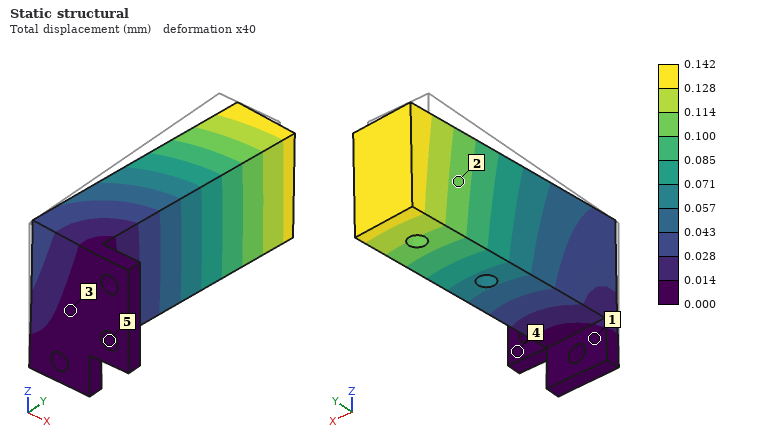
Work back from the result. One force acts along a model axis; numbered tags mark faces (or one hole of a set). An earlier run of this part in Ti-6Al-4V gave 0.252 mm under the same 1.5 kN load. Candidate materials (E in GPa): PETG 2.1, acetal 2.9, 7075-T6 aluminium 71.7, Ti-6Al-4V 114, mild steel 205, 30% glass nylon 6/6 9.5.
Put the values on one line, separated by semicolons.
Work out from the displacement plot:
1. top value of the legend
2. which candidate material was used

0.142 mm; mild steel
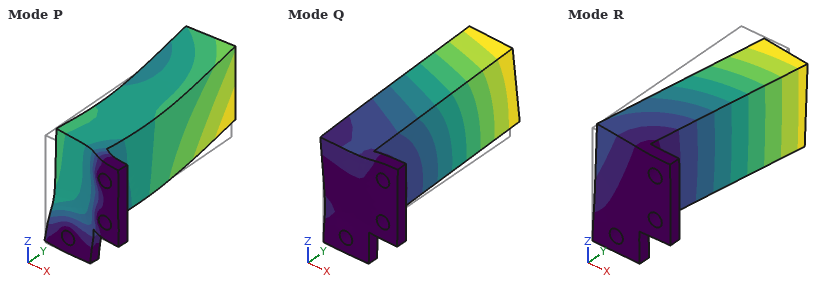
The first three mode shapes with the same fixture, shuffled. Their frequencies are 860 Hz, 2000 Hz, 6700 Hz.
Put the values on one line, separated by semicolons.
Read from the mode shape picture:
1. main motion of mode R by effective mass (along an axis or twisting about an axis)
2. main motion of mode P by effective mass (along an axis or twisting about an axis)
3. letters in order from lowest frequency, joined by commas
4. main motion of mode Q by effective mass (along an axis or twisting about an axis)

along X; along Y; R, Q, P; along Z
